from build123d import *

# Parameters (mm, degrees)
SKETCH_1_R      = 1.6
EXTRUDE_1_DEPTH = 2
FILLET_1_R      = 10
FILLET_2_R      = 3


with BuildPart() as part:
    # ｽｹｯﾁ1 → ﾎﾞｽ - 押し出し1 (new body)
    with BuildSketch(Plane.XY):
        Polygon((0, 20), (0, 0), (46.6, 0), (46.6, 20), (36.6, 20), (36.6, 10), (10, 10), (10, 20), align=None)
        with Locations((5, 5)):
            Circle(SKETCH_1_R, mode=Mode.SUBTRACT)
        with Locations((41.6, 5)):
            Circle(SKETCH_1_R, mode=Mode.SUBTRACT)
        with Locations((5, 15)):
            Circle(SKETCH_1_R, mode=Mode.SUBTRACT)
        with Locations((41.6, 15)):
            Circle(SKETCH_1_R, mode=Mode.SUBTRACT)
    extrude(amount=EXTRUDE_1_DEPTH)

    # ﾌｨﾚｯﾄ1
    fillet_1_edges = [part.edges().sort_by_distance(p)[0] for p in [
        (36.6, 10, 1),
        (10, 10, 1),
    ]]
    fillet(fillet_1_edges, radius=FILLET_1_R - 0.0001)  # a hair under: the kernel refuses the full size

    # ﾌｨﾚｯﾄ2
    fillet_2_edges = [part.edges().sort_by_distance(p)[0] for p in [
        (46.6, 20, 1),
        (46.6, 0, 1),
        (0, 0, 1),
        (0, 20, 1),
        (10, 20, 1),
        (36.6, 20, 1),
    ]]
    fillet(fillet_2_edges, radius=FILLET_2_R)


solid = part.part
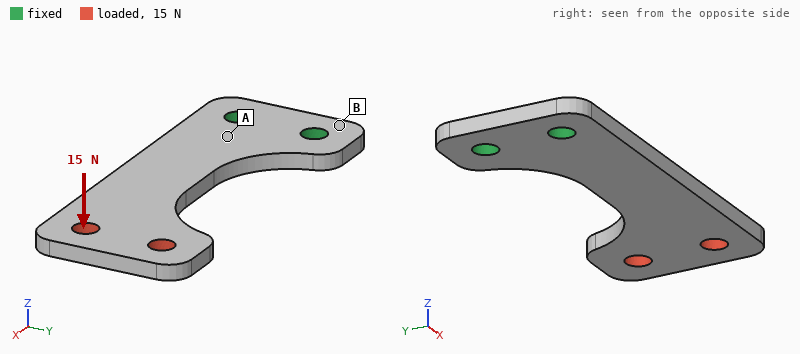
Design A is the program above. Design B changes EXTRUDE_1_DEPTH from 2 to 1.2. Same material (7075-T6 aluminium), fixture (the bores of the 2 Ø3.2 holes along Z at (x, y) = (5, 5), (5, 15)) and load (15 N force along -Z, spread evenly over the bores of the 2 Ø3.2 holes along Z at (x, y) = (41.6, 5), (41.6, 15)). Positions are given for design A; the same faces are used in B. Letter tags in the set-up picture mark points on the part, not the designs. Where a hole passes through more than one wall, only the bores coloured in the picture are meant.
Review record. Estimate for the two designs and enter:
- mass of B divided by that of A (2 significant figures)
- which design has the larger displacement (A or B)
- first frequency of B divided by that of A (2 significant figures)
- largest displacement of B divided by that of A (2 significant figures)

0.60
B
0.61
4.5
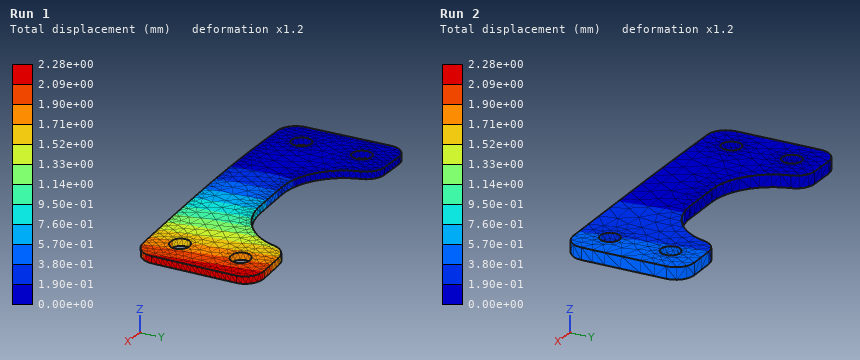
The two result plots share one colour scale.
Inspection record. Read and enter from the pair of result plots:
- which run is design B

Run 1
